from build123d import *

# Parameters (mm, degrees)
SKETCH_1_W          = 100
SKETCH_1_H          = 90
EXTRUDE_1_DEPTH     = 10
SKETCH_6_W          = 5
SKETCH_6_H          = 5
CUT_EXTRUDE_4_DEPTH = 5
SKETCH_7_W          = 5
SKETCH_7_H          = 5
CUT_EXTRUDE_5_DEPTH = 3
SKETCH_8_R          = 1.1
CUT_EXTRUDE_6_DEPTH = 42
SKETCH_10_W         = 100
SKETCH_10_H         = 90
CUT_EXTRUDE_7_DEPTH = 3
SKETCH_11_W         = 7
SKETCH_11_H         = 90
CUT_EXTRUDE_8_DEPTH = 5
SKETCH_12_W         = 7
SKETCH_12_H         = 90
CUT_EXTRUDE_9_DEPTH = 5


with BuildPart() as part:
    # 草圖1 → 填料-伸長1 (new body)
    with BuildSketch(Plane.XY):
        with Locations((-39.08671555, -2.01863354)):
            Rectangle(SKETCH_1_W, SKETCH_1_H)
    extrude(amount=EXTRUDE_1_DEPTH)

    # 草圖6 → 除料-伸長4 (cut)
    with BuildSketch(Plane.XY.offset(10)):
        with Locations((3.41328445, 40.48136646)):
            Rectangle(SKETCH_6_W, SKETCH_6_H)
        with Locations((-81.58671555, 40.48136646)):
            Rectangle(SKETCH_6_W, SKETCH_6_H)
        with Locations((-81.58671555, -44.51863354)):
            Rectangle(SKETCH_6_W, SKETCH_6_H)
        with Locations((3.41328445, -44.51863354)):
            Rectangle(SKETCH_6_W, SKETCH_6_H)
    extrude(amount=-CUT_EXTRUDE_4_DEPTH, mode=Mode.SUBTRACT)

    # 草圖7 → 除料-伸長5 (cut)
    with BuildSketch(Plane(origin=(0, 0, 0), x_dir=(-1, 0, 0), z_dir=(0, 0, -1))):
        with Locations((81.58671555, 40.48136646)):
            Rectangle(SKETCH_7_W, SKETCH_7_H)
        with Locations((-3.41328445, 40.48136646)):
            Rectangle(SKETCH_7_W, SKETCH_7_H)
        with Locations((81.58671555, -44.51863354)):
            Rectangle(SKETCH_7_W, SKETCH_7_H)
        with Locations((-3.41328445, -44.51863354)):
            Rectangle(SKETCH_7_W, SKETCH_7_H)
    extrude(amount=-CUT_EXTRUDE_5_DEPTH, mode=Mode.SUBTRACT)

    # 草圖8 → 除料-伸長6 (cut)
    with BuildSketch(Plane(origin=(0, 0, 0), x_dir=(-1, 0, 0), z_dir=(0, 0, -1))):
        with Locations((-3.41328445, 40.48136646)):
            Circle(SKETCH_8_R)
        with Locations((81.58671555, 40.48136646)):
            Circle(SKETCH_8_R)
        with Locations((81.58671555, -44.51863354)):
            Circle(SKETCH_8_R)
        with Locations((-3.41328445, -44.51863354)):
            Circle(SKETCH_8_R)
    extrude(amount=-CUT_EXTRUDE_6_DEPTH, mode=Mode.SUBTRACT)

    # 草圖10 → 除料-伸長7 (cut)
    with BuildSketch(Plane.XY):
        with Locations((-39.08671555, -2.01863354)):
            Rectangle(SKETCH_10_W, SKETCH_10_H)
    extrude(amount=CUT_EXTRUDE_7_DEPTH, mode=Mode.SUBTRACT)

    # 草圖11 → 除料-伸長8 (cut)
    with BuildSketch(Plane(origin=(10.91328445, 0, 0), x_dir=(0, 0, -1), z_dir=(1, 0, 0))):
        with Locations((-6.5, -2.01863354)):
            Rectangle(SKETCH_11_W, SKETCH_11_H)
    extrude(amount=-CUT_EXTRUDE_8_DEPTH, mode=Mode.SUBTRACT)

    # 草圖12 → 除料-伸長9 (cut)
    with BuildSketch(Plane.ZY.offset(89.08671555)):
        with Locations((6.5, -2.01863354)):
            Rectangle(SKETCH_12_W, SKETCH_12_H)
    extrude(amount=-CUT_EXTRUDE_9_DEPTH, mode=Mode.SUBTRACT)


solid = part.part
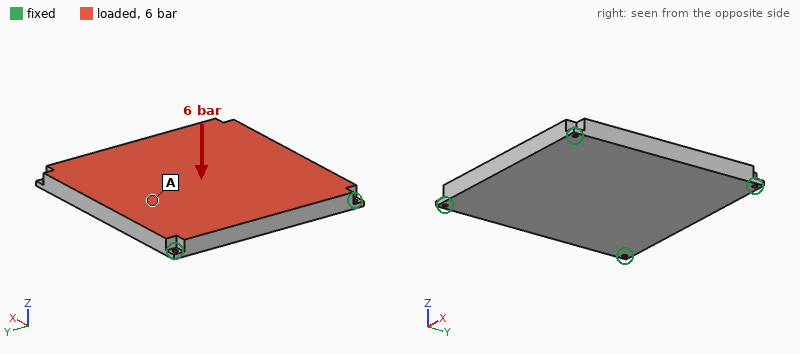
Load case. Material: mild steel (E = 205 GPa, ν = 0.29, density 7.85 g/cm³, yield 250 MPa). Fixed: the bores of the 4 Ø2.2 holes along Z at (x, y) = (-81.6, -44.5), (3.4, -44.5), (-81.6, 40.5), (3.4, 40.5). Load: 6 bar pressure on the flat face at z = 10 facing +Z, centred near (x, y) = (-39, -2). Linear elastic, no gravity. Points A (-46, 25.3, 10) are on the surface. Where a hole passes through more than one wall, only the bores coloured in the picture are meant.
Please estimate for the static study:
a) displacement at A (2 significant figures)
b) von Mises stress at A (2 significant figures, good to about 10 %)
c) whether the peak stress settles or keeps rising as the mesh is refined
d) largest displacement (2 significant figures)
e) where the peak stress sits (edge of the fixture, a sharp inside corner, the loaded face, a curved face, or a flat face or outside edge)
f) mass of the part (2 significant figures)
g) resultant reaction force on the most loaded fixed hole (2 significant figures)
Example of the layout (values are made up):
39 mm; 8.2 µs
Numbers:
68 µm; 48 MPa; keeps rising; 84 µm; edge of the fixture; 440 g; 2.7 kN
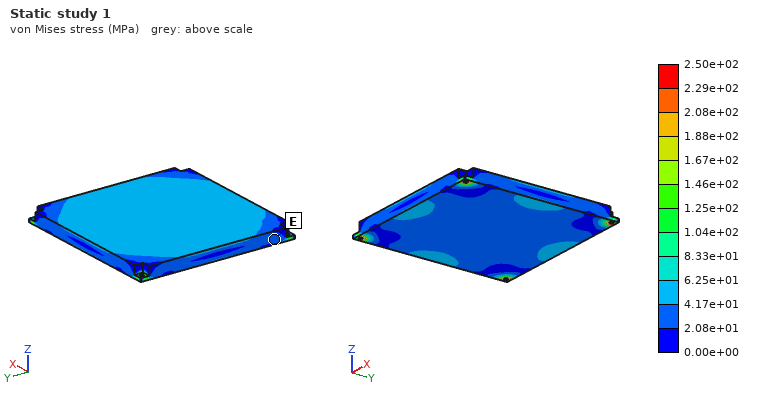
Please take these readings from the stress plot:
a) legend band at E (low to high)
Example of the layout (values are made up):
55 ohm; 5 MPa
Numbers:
2.08e+01 to 4.17e+01 MPa
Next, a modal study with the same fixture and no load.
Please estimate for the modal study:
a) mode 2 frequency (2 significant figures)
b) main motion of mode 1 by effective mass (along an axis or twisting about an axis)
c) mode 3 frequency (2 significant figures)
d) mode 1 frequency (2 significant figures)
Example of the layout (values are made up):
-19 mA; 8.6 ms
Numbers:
3900 Hz; along Z; 3900 Hz; 2100 Hz
